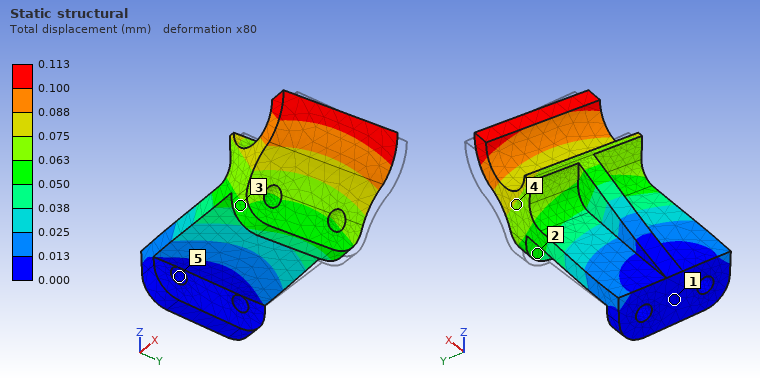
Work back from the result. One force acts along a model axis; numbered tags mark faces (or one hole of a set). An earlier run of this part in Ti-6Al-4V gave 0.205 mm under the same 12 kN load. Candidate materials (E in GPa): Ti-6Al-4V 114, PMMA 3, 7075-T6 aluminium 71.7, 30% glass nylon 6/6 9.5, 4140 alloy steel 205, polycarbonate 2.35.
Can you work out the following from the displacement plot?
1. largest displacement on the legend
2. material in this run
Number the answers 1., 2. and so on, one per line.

1. 0.113 mm
2. 4140 alloy steel
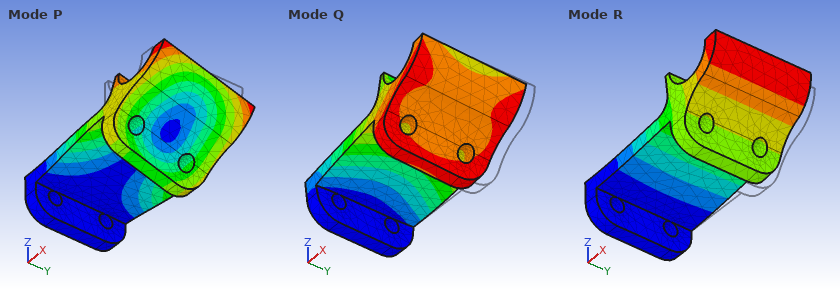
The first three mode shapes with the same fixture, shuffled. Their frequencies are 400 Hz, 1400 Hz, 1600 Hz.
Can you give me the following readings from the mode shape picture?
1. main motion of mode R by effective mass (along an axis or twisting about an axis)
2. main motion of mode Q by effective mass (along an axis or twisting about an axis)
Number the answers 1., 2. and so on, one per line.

1. along Z
2. along Y
